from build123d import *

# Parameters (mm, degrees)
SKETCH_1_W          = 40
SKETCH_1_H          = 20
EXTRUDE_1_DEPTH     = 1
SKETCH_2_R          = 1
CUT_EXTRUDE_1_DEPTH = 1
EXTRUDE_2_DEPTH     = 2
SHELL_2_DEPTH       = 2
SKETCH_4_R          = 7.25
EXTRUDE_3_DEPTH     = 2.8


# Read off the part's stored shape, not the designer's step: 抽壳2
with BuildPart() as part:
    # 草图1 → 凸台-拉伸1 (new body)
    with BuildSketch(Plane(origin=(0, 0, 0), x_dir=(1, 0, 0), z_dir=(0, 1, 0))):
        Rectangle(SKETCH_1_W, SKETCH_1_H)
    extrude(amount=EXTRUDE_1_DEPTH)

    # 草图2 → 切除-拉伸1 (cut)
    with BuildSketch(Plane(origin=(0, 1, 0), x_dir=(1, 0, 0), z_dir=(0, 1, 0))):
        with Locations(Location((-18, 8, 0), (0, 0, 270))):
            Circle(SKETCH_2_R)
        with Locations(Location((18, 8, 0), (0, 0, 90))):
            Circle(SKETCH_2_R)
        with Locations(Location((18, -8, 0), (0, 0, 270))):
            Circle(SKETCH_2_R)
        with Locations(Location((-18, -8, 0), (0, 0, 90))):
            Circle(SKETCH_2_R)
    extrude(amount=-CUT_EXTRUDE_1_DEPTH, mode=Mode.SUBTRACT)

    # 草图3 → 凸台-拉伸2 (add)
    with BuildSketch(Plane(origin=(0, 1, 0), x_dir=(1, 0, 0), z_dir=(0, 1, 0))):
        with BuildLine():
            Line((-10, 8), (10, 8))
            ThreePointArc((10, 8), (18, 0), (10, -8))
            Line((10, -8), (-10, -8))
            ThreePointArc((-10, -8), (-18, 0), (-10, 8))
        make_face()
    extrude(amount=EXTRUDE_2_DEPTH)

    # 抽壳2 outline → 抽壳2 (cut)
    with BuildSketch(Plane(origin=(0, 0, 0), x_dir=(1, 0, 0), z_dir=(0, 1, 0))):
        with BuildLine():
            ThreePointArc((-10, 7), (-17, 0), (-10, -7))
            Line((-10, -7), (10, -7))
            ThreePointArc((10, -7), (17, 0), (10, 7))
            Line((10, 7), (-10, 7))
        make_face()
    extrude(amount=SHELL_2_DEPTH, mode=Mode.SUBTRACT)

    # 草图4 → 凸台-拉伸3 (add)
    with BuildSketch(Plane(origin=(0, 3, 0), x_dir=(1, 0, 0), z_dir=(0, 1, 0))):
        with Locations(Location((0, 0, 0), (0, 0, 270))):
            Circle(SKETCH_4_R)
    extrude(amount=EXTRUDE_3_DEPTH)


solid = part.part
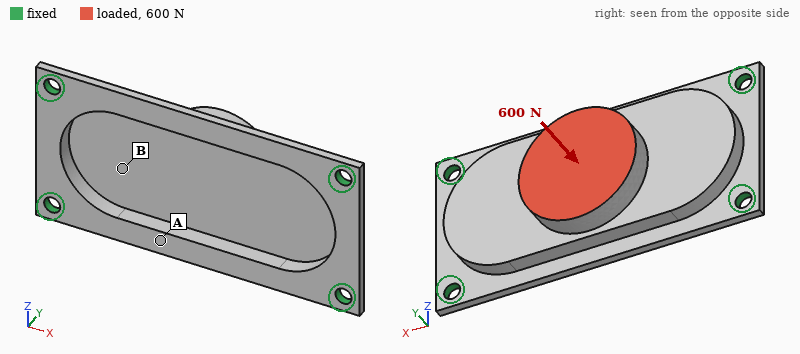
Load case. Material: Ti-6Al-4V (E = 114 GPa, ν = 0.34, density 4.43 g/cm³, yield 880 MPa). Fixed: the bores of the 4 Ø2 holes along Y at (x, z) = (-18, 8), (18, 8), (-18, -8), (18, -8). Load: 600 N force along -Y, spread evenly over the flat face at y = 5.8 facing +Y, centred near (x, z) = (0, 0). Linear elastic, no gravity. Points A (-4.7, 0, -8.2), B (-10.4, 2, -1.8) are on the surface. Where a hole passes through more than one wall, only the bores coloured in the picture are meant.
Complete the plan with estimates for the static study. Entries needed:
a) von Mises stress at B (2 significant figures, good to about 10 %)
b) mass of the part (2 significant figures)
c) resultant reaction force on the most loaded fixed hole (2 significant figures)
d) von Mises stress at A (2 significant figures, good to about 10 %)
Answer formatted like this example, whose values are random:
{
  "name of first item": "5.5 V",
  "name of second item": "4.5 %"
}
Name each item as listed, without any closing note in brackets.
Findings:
{
  "von Mises stress at B": "53 MPa",
  "mass of the part": "6.3 g",
  "resultant reaction force on the most loaded fixed hole": "450 N",
  "von Mises stress at A": "100 MPa"
}
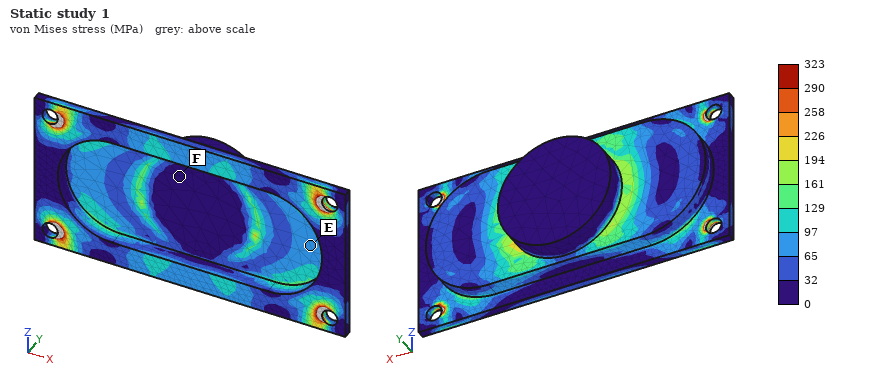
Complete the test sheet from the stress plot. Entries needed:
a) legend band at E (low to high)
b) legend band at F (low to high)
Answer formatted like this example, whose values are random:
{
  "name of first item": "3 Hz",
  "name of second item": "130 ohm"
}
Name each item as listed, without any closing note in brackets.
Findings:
{
  "legend band at E": "65 to 97 MPa",
  "legend band at F": "0 to 32 MPa"
}
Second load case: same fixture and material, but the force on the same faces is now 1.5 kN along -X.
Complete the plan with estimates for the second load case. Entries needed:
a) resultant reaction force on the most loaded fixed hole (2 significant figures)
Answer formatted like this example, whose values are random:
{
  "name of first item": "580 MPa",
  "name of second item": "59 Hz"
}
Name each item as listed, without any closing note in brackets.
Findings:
{
  "resultant reaction force on the most loaded fixed hole": "400 N"
}
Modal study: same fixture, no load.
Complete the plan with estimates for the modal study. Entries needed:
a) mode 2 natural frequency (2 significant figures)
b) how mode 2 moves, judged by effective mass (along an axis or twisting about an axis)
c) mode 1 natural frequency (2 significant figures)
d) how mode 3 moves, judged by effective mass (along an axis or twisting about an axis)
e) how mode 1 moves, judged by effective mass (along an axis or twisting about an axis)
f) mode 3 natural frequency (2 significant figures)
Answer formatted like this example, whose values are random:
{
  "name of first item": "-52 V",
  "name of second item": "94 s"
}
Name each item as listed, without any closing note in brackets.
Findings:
{
  "mode 2 natural frequency": "8800 Hz",
  "how mode 2 moves, judged by effective mass": "twisting about X",
  "mode 1 natural frequency": "7100 Hz",
  "how mode 3 moves, judged by effective mass": "twisting about Z",
  "how mode 1 moves, judged by effective mass": "along Y",
  "mode 3 natural frequency": "16 kHz"
}
